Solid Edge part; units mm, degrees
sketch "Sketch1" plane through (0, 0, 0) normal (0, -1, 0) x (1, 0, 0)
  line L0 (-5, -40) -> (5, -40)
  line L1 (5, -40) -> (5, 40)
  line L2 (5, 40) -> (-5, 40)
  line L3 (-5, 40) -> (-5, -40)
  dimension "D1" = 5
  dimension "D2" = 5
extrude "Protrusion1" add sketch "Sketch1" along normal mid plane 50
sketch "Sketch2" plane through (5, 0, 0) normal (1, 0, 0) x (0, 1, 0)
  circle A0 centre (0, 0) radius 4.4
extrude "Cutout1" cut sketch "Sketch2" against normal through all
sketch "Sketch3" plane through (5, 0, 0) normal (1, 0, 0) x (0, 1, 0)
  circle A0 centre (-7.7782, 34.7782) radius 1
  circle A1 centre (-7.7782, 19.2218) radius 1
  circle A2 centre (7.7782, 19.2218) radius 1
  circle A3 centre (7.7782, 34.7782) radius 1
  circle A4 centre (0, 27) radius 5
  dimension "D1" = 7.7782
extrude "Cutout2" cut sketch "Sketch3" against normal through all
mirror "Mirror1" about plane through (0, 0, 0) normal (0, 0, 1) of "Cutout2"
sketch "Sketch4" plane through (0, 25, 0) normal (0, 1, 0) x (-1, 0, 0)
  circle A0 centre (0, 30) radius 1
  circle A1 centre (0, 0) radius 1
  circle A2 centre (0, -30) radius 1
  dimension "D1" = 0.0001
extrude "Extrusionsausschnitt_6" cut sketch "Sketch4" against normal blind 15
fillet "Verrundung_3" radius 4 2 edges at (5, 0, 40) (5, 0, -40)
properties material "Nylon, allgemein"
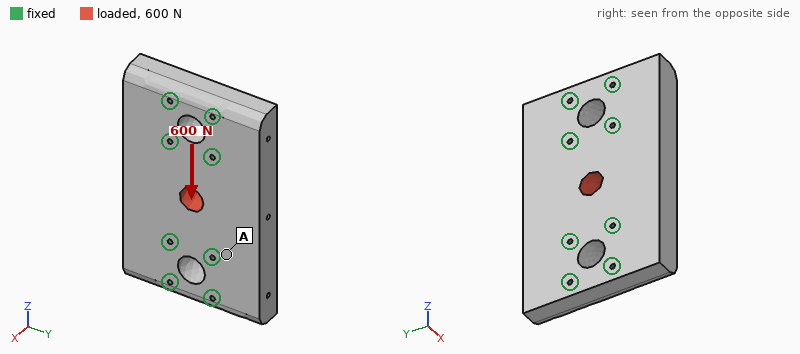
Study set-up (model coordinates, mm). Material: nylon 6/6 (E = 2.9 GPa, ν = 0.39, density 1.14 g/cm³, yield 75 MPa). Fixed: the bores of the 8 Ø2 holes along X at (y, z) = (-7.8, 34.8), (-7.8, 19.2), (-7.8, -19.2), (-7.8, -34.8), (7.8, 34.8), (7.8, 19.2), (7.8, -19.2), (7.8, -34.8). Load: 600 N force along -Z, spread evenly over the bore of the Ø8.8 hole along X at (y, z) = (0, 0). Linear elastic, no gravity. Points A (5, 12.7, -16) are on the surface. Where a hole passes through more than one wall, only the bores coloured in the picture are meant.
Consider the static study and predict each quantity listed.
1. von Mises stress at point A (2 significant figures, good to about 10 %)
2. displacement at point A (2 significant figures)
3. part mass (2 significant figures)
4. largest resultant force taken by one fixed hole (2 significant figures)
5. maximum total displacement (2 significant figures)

0.43 MPa
2.8 µm
42 g
140 N
11 µm
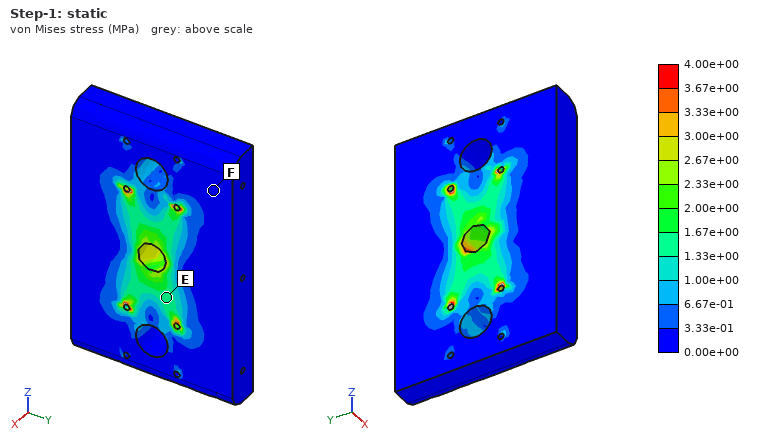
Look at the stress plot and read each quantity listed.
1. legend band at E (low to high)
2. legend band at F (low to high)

1.33e+00 to 1.67e+00 MPa
0.00e+00 to 3.33e-01 MPa
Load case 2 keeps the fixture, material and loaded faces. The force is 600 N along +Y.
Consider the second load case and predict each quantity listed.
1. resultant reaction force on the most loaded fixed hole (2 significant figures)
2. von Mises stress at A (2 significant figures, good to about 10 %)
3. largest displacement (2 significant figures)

160 N
1.3 MPa
18 µm
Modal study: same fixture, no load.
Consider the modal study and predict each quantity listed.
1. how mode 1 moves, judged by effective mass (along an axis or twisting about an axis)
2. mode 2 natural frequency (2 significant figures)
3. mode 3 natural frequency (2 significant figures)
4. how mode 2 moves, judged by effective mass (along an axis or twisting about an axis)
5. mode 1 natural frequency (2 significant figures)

twisting about Z
4900 Hz
6500 Hz
along X
4600 Hz
